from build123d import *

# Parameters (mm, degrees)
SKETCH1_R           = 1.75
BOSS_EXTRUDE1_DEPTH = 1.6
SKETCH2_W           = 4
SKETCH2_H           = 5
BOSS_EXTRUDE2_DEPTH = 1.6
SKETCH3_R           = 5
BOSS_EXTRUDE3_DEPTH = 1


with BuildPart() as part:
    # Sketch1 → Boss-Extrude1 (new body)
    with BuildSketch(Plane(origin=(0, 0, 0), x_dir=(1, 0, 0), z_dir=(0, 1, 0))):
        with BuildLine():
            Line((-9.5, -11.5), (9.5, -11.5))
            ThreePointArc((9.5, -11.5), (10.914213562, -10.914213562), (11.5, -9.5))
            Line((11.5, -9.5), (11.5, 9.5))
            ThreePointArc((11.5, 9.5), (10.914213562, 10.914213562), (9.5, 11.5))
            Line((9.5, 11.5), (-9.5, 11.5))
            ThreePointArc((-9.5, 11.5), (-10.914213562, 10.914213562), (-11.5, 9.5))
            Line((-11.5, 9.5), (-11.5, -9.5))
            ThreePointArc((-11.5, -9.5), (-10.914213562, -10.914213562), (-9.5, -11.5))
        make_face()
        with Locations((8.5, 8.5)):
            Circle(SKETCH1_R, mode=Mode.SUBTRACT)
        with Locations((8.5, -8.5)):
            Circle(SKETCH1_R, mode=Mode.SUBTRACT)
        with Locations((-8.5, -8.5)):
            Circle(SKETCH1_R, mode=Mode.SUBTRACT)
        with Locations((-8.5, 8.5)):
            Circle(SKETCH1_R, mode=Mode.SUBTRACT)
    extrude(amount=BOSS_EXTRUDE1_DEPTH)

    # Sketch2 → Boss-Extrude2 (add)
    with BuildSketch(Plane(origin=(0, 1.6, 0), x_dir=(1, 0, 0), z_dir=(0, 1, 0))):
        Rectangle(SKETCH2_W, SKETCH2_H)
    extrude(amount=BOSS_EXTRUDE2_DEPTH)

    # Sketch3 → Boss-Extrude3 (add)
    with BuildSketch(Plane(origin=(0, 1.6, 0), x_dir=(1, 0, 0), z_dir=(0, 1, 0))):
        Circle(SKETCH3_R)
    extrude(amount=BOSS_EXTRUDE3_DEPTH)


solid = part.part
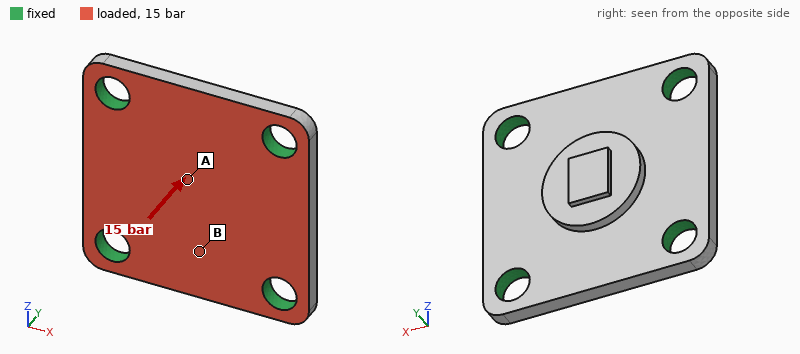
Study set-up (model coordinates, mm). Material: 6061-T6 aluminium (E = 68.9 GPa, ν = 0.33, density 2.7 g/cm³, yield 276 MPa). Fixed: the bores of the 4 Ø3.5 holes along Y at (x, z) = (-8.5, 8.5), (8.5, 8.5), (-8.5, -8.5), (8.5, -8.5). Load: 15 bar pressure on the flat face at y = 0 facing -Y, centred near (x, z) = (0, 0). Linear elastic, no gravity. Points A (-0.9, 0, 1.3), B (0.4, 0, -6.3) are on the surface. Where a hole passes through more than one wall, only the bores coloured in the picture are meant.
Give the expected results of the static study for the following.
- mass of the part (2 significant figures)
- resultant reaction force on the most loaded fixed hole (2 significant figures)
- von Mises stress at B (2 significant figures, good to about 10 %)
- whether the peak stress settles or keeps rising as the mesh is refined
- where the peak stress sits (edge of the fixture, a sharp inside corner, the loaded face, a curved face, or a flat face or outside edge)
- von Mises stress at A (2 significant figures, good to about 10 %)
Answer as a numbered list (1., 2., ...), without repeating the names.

1. 2.3 g
2. 180 N
3. 27 MPa
4. keeps rising
5. edge of the fixture
6. 12 MPa
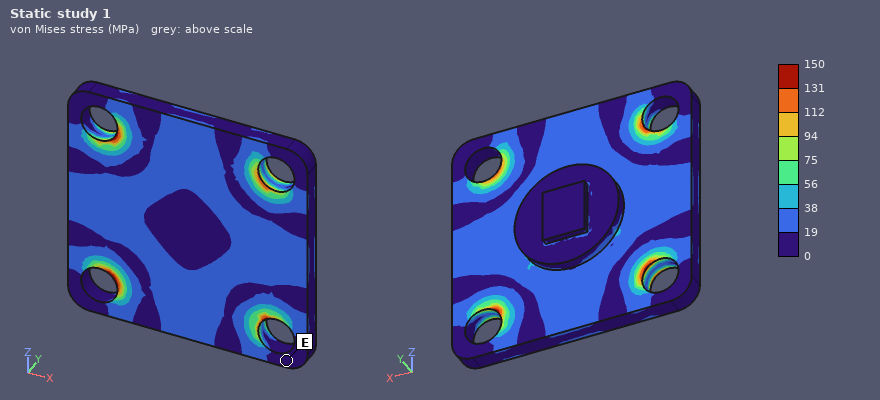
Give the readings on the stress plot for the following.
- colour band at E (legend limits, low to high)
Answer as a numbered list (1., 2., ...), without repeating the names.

1. 0 to 19 MPa
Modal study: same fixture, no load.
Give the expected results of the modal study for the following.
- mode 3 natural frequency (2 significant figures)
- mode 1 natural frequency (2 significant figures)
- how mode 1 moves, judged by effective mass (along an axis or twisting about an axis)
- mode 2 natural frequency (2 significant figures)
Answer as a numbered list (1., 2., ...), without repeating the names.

1. 40 kHz
2. 26 kHz
3. along Y
4. 40 kHz
